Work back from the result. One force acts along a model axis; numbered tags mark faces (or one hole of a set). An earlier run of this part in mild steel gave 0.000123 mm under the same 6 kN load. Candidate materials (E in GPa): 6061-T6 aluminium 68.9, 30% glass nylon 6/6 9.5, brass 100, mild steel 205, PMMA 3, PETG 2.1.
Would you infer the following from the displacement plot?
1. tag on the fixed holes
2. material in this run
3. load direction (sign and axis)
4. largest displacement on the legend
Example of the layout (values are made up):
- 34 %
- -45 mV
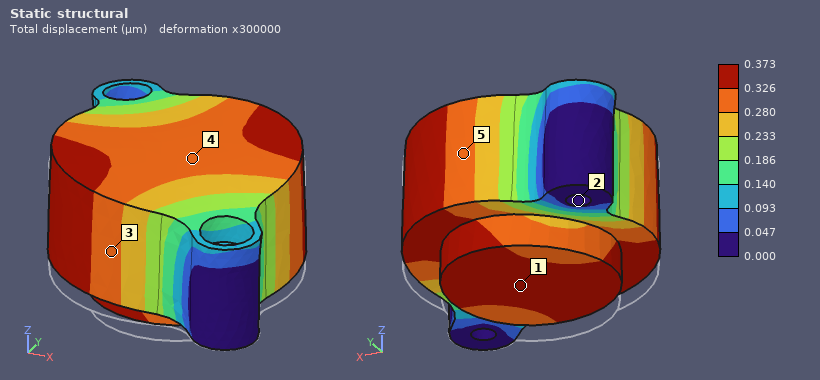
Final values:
- 2
- 6061-T6 aluminium
- +Z
- 0.373 µm
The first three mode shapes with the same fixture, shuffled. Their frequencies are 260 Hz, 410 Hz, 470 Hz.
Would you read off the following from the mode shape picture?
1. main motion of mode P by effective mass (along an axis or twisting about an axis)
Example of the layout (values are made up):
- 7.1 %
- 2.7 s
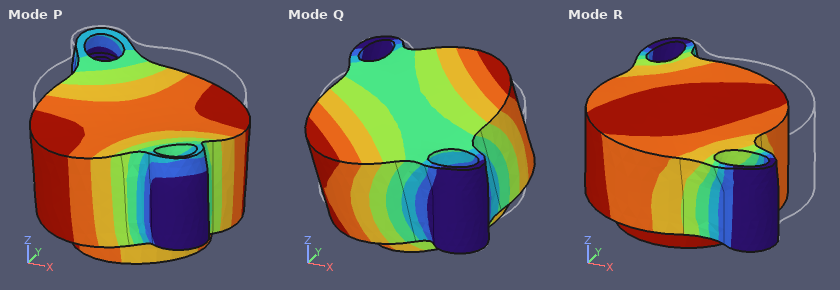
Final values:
- along Z
